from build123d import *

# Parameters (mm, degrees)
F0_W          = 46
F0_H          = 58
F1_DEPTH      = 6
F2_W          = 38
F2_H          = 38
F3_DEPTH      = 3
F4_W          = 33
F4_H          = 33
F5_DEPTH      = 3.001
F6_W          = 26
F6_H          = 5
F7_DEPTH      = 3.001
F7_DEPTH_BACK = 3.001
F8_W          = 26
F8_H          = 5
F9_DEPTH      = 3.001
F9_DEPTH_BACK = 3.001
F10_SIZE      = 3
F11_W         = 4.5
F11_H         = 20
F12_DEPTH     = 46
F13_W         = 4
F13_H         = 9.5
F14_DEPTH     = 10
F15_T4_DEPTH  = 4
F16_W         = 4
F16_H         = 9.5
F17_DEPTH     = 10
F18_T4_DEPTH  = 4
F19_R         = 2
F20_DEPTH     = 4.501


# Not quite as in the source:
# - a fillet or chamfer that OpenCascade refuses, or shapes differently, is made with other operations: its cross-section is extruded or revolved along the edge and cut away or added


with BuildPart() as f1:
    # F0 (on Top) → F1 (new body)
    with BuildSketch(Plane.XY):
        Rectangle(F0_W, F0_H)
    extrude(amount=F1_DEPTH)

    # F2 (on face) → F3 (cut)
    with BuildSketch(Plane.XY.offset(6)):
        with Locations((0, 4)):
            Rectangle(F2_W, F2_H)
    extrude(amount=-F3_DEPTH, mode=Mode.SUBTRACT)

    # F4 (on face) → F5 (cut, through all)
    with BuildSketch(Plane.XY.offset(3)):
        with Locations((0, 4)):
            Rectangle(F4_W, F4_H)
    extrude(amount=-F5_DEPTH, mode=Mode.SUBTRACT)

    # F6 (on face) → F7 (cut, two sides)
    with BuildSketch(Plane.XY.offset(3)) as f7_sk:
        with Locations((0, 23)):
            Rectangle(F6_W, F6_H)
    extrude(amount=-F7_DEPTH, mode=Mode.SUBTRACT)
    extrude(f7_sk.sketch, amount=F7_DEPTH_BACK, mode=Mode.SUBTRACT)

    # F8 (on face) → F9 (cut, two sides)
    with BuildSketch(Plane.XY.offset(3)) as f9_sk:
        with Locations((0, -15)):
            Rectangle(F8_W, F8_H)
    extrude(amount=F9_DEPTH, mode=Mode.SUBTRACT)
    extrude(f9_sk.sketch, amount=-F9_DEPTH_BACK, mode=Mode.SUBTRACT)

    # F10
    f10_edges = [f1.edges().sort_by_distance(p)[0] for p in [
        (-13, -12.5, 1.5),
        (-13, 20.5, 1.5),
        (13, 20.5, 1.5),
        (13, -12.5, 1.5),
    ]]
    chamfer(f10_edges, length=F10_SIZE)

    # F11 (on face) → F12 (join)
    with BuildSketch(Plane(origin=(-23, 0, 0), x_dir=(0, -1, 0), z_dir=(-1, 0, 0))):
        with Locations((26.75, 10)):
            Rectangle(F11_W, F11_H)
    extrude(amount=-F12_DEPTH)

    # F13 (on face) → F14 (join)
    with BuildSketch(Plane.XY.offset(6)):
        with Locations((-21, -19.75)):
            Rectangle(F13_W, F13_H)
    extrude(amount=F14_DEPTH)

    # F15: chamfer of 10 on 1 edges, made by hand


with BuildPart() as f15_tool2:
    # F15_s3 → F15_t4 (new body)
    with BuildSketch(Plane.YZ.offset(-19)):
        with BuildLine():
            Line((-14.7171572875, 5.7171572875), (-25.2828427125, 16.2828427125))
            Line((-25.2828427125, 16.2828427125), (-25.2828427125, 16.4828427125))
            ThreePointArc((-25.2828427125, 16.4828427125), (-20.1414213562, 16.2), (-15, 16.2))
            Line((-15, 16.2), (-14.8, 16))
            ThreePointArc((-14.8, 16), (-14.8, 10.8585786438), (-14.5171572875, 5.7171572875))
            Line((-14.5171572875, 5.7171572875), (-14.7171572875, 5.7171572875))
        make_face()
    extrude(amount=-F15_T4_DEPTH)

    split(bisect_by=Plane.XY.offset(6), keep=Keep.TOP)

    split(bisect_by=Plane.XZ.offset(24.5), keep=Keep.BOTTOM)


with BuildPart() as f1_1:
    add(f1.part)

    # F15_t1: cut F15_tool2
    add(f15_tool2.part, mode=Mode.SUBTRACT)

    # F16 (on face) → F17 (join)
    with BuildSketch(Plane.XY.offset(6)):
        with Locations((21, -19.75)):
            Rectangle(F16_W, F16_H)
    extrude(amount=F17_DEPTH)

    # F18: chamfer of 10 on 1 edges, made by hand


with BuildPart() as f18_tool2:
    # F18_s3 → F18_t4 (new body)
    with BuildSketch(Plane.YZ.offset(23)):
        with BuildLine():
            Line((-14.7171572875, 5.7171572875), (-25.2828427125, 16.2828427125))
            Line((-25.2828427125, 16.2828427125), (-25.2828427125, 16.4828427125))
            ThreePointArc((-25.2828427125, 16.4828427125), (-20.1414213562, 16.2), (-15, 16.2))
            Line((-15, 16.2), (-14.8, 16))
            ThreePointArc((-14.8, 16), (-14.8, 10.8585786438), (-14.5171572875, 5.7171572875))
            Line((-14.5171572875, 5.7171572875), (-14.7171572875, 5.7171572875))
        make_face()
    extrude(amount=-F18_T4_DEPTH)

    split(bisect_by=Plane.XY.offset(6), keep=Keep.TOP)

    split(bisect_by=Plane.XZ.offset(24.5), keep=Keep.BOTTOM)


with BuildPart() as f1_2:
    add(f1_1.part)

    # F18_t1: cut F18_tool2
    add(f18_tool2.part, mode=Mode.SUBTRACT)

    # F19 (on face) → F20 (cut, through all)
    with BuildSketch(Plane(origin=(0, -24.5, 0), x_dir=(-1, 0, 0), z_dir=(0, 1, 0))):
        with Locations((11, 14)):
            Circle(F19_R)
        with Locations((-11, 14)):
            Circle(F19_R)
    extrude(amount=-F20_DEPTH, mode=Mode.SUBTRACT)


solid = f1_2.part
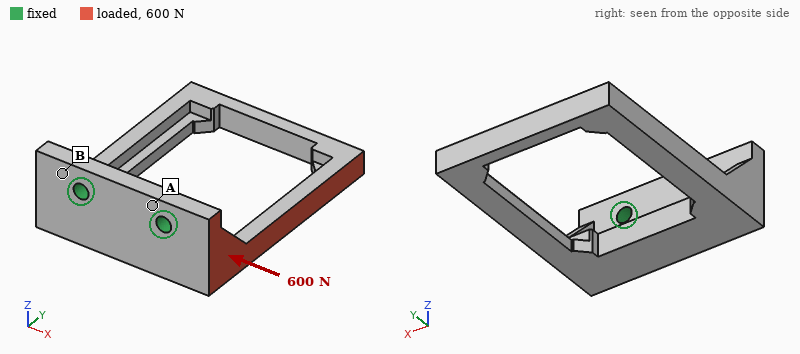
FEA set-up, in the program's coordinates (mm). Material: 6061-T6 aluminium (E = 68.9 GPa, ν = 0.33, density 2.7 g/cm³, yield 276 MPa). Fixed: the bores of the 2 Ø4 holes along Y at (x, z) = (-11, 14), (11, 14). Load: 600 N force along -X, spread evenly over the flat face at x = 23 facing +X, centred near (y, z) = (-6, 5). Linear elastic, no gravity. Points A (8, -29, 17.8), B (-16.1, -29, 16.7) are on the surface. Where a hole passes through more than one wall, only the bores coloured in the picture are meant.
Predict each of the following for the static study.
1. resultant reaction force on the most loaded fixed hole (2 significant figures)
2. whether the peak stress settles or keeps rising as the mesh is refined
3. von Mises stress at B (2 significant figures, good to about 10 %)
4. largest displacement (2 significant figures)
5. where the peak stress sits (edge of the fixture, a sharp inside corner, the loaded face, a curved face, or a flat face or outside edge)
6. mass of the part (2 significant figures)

580 N
keeps rising
21 MPa
0.25 mm
a sharp inside corner
28 g
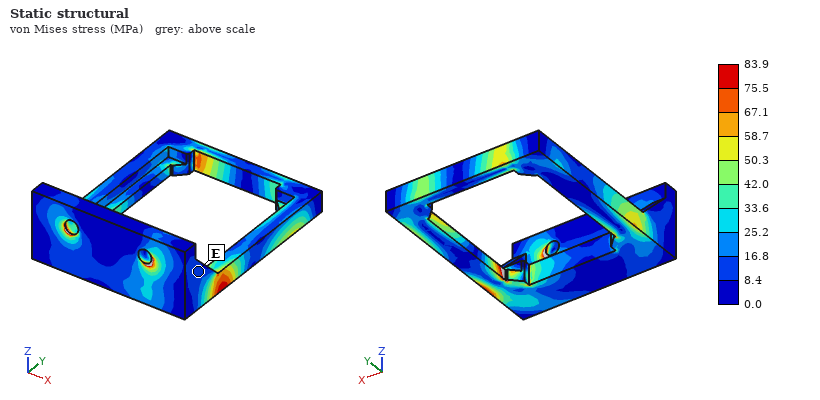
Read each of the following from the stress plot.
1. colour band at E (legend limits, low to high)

8.4 to 16.8 MPa
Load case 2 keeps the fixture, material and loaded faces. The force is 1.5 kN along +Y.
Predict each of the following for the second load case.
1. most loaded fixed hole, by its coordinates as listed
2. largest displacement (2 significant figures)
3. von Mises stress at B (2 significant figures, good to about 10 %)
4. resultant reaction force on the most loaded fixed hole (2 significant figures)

(11, 14)
0.32 mm
28 MPa
1.9 kN
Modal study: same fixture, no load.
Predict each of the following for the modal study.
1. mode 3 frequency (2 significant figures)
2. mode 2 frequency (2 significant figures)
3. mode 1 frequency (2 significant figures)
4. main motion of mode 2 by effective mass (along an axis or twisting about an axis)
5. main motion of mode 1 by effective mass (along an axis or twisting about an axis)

2700 Hz
1900 Hz
1200 Hz
along X
along Z
